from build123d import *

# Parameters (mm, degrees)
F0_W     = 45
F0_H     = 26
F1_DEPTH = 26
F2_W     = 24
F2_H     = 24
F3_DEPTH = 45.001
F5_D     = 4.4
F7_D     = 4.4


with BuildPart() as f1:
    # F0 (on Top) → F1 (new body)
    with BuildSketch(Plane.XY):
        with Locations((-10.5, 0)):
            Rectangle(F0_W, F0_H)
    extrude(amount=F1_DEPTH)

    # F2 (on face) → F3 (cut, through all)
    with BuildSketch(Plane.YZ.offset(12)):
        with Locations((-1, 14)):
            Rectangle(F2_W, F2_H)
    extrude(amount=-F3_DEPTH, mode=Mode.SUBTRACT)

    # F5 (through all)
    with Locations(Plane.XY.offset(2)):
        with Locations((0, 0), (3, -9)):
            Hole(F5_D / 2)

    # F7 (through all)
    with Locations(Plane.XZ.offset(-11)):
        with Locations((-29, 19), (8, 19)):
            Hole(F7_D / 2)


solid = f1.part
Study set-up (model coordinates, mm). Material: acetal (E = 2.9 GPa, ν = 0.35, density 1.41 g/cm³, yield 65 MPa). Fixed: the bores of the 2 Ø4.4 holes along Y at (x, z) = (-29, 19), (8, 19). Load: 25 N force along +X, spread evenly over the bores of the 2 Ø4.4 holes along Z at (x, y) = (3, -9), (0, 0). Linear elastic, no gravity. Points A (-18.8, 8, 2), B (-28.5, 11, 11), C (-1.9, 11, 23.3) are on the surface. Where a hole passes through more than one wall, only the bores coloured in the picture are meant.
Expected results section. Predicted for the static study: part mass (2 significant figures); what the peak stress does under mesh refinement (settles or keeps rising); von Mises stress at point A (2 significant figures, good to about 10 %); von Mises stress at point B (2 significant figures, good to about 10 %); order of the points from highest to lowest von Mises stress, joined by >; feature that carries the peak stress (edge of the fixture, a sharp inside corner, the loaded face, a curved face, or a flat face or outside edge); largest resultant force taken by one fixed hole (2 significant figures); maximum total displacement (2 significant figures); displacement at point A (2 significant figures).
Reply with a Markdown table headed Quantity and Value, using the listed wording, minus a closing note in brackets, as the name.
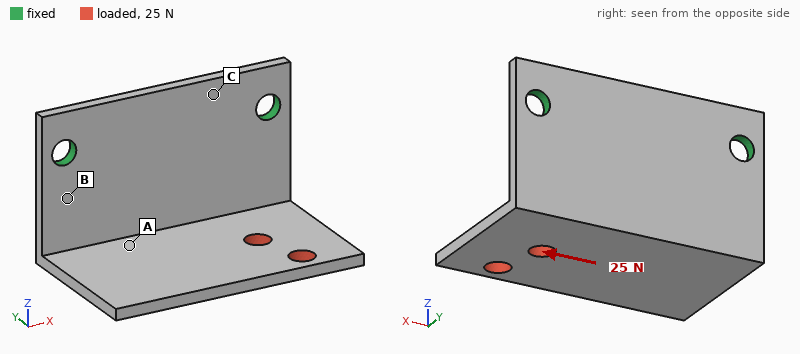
| Quantity | Value |
|---|---|
| part mass | 6.2 g |
| what the peak stress does under mesh refinement | keeps rising |
| von Mises stress at point A | 3.5 MPa |
| von Mises stress at point B | 5.8 MPa |
| order of the points from highest to lowest von Mises stress, joined by > | B > A > C |
| feature that carries the peak stress | edge of the fixture |
| largest resultant force taken by one fixed hole | 21 N |
| maximum total displacement | 0.59 mm |
| displacement at point A | 0.14 mm |
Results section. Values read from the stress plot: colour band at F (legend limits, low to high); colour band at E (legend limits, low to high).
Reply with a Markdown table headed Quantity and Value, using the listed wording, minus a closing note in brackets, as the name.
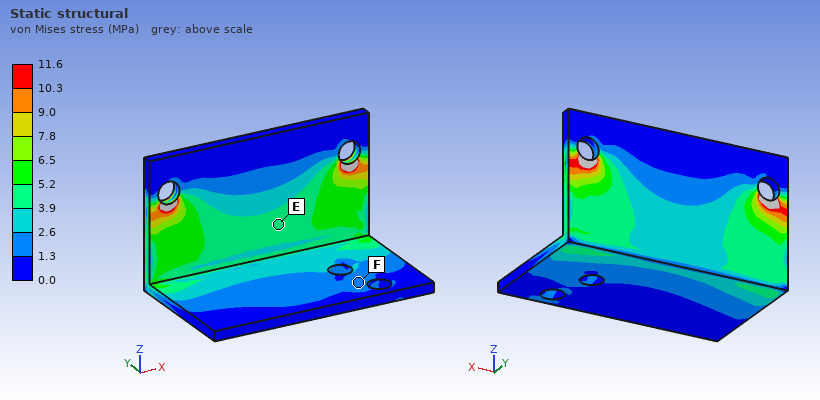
| Quantity | Value |
|---|---|
| colour band at F | 1.3 to 2.6 MPa |
| colour band at E | 3.9 to 5.2 MPa |
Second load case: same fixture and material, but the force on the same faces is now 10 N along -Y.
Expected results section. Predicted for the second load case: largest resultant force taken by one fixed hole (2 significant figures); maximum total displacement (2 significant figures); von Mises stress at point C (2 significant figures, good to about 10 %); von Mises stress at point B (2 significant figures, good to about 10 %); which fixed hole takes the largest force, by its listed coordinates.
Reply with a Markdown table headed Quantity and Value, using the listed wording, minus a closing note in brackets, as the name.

| Quantity | Value |
|---|---|
| largest resultant force taken by one fixed hole | 8.4 N |
| maximum total displacement | 0.67 mm |
| von Mises stress at point C | 1.8 MPa |
| von Mises stress at point B | 2.9 MPa |
| which fixed hole takes the largest force, by its listed coordinates | (8, 19) |
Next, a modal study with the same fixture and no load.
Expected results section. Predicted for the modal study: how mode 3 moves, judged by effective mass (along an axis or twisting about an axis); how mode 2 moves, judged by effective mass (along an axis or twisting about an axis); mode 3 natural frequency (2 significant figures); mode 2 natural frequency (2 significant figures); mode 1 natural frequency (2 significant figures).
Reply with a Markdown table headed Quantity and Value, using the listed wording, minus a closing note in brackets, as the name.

| Quantity | Value |
|---|---|
| how mode 3 moves, judged by effective mass | along Y |
| how mode 2 moves, judged by effective mass | along X |
| mode 3 natural frequency | 920 Hz |
| mode 2 natural frequency | 670 Hz |
| mode 1 natural frequency | 340 Hz |
